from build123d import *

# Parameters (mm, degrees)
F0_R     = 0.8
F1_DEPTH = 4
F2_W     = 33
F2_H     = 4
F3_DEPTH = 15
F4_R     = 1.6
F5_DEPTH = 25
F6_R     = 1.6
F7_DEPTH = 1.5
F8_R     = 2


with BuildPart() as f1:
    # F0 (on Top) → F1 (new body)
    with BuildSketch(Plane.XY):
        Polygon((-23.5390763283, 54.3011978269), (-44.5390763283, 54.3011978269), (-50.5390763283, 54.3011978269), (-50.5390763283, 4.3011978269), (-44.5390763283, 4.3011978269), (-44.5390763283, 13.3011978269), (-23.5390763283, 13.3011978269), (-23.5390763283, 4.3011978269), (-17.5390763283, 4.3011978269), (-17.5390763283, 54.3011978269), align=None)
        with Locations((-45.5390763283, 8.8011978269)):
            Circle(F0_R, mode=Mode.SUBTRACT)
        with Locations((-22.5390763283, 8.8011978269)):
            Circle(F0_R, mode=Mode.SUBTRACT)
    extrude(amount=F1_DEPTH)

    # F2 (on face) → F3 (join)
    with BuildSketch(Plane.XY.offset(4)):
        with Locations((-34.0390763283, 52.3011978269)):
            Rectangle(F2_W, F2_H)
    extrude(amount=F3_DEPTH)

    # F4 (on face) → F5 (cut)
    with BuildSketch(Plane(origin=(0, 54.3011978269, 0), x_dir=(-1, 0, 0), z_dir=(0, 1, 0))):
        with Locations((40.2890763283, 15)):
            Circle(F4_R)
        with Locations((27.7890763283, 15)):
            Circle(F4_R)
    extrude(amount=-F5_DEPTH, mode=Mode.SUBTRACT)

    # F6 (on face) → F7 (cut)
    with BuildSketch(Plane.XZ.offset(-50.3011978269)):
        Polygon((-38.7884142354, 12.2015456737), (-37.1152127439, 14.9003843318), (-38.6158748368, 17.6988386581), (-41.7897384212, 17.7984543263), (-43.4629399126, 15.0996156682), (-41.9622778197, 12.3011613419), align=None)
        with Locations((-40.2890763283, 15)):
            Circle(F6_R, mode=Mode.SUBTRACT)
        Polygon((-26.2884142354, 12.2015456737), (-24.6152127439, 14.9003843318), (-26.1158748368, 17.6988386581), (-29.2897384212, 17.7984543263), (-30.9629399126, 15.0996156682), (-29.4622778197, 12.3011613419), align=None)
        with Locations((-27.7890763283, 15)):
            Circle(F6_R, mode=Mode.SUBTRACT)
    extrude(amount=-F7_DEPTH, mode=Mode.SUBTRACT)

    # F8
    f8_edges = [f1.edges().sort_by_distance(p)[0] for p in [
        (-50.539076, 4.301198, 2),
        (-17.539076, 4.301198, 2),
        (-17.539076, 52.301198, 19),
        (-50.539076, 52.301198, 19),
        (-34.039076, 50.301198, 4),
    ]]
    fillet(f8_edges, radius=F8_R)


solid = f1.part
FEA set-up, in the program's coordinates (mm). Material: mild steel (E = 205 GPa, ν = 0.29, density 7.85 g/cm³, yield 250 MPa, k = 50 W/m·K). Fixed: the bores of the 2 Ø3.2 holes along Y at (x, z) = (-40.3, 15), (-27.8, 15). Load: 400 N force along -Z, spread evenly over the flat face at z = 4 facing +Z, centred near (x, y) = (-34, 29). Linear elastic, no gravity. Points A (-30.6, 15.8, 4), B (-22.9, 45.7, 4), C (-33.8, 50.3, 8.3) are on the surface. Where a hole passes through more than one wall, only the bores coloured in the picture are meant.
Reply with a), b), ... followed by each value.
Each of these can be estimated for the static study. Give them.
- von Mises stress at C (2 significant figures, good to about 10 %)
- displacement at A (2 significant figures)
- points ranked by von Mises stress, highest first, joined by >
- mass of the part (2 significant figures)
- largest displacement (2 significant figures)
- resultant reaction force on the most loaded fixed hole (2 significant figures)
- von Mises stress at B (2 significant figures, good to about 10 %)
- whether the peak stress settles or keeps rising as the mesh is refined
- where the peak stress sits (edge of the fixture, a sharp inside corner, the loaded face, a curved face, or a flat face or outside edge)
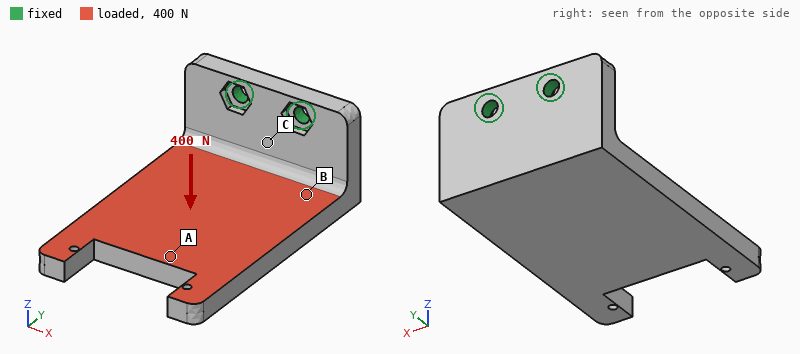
a) 120 MPa
b) 0.24 mm
c) C > B > A
d) 60 g
e) 0.33 mm
f) 200 N
g) 71 MPa
h) keeps rising
i) edge of the fixture
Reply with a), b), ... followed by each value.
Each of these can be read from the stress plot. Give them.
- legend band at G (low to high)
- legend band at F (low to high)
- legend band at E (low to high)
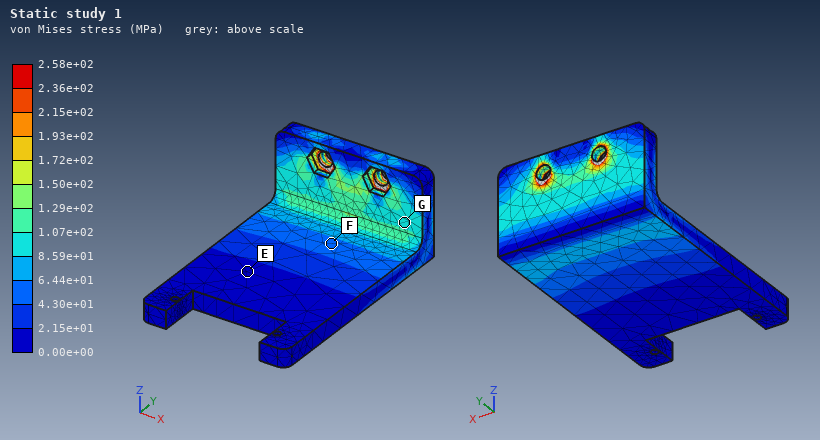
a) 8.59e+01 to 1.07e+02 MPa
b) 4.30e+01 to 6.44e+01 MPa
c) 0.00e+00 to 2.15e+01 MPa
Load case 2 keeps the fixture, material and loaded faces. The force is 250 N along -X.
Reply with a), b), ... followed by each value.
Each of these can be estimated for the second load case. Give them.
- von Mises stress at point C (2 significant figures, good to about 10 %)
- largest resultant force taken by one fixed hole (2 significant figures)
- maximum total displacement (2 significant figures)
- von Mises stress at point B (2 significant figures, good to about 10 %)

a) 49 MPa
b) 440 N
c) 49 µm
d) 23 MPa
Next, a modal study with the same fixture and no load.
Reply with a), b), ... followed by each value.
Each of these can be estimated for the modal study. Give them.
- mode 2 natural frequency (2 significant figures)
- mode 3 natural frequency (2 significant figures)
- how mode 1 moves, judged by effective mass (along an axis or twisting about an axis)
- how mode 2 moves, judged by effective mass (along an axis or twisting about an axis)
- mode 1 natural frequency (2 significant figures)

a) 2300 Hz
b) 4500 Hz
c) along Z
d) along X
e) 1100 Hz
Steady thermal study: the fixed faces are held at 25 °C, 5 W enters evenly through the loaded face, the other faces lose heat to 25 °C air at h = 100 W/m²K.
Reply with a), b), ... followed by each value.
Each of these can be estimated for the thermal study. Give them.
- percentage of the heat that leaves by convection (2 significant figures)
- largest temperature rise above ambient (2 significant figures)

a) 54 %
b) 14 K
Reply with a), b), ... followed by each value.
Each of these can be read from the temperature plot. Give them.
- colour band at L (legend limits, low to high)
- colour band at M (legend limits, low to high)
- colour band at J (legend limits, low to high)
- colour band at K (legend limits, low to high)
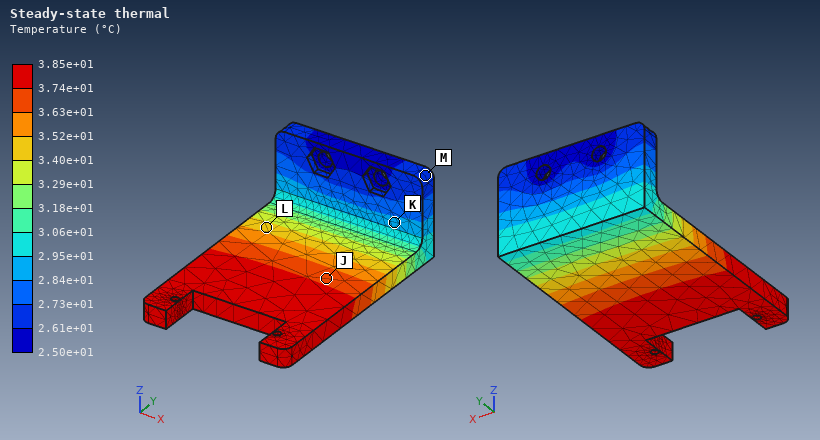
a) 3.40e+01 to 3.52e+01 °C
b) 2.61e+01 to 2.73e+01 °C
c) 3.63e+01 to 3.74e+01 °C
d) 2.84e+01 to 2.95e+01 °C
